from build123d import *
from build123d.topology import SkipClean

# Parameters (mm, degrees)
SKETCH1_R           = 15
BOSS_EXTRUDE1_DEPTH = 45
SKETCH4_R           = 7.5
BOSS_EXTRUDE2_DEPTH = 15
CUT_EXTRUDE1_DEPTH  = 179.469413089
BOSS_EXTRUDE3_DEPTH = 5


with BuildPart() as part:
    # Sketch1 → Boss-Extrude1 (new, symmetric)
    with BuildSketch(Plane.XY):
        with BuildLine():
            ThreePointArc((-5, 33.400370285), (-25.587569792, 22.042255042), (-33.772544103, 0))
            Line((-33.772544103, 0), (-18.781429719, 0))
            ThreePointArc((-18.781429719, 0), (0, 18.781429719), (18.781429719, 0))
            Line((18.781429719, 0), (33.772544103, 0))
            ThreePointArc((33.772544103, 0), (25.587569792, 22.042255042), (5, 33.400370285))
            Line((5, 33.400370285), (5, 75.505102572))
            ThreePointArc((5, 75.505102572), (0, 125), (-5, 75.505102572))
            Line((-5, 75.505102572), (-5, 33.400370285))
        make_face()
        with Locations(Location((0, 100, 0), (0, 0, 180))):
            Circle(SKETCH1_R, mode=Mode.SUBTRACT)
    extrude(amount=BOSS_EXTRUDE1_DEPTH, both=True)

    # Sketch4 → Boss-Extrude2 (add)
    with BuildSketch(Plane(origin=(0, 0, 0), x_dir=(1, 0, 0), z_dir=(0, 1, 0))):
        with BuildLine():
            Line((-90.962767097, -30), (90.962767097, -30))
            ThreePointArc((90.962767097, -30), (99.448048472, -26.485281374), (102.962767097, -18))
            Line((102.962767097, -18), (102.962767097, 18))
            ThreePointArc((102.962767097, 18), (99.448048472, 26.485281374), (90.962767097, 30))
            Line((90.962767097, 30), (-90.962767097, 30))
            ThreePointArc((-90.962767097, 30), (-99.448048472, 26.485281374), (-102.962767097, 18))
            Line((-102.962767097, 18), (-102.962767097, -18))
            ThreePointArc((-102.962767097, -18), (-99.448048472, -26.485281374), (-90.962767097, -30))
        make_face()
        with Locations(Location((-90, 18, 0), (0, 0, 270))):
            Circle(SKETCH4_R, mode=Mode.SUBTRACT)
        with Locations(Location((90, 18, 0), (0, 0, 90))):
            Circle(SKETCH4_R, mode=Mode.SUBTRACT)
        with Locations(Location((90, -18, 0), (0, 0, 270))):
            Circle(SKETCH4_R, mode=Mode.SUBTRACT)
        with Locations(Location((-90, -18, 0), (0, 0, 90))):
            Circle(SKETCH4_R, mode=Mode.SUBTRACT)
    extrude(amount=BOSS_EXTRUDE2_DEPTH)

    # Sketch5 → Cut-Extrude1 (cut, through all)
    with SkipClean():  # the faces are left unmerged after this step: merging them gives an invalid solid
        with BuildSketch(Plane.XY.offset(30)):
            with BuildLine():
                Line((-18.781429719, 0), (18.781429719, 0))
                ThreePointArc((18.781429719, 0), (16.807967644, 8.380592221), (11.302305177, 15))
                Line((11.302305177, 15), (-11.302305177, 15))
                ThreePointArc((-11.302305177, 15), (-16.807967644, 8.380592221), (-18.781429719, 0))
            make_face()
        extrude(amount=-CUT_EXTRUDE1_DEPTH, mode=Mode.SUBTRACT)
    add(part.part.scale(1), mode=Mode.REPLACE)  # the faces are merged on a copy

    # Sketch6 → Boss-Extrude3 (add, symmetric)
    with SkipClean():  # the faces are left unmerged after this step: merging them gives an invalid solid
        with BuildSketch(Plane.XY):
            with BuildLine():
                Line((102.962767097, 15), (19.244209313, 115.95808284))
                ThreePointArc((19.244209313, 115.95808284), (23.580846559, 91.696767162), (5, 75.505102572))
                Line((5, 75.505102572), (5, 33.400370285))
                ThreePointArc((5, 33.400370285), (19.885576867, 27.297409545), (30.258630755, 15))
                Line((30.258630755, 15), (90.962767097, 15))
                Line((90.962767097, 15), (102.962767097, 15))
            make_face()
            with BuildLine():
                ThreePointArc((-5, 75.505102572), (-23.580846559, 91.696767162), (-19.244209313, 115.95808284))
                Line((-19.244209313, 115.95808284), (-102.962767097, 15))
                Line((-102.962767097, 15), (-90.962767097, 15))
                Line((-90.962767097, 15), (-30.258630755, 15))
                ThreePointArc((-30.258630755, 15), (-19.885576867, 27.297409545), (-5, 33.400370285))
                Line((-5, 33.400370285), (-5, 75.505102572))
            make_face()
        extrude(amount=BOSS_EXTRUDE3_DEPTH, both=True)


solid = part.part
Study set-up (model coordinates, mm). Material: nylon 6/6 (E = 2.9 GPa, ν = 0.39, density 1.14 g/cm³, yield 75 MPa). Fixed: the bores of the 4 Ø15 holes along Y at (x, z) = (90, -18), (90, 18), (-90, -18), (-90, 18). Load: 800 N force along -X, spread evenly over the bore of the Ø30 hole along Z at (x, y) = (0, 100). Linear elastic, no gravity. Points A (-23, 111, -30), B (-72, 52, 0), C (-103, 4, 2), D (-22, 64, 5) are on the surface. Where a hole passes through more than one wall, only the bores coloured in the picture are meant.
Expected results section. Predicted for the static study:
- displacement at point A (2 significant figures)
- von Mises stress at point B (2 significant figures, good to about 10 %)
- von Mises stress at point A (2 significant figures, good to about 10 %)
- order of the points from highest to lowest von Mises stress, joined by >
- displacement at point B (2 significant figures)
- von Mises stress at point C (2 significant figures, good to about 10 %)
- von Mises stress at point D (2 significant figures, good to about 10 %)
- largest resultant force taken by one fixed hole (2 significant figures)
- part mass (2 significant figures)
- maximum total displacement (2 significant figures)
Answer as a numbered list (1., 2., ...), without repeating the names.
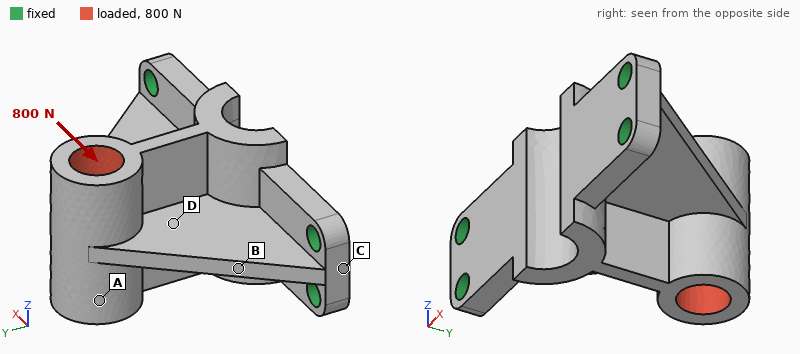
1. 0.11 mm
2. 1.8 MPa
3. 0.32 MPa
4. B > D > C > A
5. 0.030 mm
6. 0.58 MPa
7. 0.90 MPa
8. 310 N
9. 540 g
10. 0.12 mm
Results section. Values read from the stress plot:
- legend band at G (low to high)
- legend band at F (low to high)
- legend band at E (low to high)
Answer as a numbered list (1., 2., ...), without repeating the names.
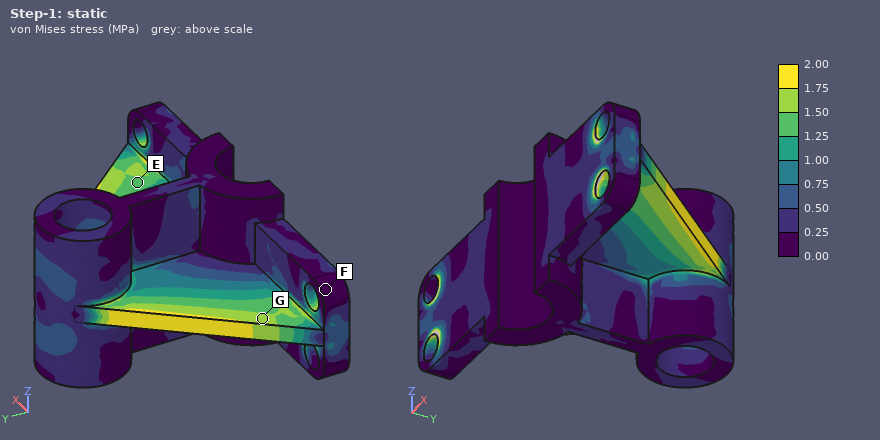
1. 1.50 to 1.75 MPa
2. 0.00 to 0.25 MPa
3. 1.25 to 1.50 MPa
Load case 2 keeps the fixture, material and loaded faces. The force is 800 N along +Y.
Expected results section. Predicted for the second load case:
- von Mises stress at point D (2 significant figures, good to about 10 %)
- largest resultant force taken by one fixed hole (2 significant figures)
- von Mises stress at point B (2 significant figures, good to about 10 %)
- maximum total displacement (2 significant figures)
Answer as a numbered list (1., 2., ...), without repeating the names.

1. 0.71 MPa
2. 300 N
3. 1.2 MPa
4. 67 µm
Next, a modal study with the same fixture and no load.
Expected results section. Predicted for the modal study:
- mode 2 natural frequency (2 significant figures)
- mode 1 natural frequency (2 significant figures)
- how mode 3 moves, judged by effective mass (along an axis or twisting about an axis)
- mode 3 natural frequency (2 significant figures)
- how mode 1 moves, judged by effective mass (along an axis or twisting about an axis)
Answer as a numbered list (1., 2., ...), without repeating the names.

1. 720 Hz
2. 230 Hz
3. along Y
4. 990 Hz
5. along Z
